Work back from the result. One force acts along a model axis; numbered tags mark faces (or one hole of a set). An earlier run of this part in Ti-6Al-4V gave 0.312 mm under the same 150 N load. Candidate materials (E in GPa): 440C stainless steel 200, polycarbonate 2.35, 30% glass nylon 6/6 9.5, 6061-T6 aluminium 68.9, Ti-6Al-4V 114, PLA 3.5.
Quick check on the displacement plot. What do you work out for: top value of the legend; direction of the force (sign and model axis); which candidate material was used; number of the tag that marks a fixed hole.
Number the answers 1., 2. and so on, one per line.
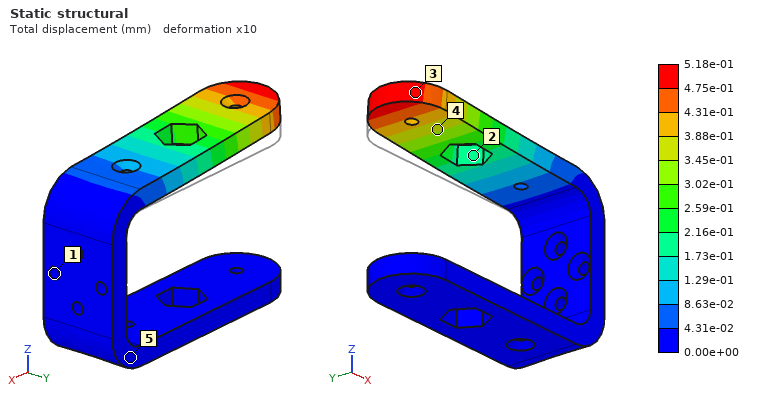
1. 5.18e-01 mm
2. +Z
3. 6061-T6 aluminium
4. 1
